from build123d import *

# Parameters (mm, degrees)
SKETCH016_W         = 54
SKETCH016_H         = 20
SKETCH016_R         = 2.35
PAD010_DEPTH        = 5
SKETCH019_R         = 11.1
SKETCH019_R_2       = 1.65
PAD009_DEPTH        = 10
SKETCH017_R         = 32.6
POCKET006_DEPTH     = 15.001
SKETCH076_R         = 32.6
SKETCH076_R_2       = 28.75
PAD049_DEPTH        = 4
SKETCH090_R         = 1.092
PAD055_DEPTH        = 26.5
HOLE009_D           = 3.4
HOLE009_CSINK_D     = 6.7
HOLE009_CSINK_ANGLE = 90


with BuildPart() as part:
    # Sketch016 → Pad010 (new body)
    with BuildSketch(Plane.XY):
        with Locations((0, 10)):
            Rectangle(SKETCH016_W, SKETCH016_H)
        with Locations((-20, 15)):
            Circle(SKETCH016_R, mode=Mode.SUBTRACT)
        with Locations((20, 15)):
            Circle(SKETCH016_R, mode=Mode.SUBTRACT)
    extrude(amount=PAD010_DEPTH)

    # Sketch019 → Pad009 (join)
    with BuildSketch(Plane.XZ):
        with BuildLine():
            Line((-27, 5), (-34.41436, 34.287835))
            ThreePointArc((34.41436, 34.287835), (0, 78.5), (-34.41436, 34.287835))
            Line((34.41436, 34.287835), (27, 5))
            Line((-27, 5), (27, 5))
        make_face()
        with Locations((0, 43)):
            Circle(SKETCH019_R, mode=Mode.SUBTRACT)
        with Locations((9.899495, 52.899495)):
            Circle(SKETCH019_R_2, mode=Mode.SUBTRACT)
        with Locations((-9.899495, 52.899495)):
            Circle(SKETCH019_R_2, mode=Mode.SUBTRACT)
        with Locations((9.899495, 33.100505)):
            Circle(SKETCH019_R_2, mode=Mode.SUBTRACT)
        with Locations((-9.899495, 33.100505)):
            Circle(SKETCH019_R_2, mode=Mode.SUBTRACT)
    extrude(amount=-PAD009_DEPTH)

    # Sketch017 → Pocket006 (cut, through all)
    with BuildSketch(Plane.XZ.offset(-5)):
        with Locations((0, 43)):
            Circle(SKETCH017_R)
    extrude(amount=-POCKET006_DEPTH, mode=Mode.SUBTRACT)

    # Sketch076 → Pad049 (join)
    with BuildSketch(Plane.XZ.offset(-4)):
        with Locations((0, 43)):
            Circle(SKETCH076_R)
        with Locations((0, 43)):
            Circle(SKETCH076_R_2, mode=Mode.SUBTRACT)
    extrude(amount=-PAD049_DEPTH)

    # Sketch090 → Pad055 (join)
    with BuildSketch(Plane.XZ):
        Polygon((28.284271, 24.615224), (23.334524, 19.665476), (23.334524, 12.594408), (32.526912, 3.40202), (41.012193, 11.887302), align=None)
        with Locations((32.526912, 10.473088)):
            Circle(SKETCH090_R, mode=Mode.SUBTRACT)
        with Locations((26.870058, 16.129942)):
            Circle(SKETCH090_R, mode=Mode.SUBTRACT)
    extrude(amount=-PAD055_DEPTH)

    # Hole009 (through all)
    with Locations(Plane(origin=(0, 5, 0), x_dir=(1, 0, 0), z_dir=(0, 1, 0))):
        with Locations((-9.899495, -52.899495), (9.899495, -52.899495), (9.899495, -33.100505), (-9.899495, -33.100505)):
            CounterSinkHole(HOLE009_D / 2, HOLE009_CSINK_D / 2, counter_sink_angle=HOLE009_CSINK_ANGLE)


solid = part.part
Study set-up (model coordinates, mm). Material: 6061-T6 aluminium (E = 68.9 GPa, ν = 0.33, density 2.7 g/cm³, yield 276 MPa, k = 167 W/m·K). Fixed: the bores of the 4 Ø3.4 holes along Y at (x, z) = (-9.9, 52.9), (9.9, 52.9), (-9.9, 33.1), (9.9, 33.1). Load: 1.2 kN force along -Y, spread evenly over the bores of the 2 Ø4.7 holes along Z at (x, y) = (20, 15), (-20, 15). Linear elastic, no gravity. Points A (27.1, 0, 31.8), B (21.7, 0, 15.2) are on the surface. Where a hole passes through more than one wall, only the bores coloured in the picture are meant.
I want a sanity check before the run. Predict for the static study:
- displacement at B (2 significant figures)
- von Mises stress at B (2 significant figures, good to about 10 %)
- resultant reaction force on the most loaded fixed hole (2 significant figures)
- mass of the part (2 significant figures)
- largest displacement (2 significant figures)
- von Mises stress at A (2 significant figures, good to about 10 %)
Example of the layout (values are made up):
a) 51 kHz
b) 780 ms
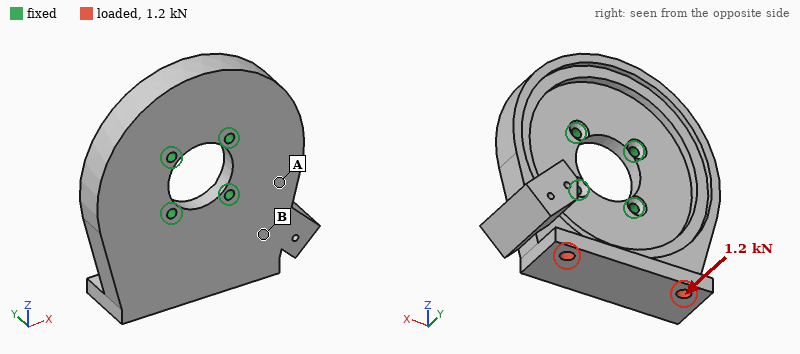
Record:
a) 0.12 mm
b) 20 MPa
c) 1.3 kN
d) 100 g
e) 0.27 mm
f) 55 MPa
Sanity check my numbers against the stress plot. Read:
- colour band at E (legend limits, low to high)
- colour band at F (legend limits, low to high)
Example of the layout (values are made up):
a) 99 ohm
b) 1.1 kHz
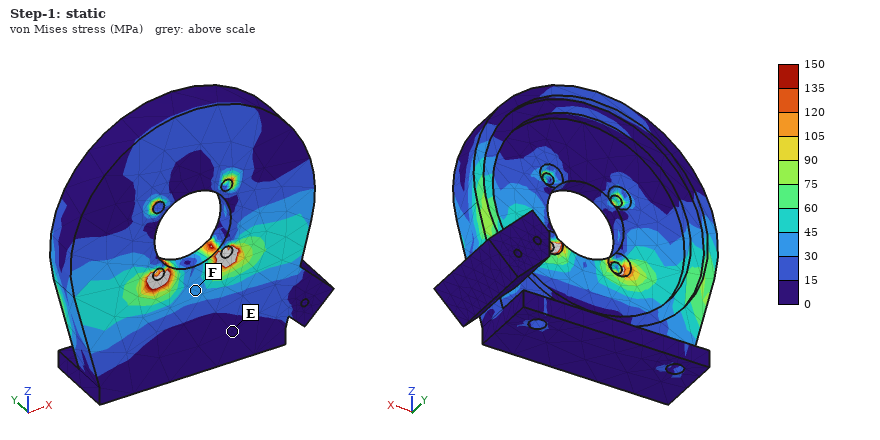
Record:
a) 0 to 15 MPa
b) 30 to 45 MPa
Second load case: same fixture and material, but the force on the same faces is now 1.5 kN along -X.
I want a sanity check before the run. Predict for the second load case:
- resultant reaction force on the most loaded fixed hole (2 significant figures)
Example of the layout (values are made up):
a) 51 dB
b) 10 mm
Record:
a) 1.6 kN
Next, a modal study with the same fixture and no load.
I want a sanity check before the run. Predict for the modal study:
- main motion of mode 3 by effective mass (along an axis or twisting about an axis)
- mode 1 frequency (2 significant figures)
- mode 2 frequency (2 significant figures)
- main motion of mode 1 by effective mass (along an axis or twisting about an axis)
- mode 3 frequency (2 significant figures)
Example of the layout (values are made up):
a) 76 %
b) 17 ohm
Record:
a) along Y
b) 1900 Hz
c) 2800 Hz
d) along Y
e) 5400 Hz
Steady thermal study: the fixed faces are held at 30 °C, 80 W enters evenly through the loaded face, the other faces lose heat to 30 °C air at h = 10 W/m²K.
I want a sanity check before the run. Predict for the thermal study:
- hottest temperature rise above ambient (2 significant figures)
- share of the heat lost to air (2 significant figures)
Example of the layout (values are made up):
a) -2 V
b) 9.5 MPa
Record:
a) 72 K
b) 4.1 %
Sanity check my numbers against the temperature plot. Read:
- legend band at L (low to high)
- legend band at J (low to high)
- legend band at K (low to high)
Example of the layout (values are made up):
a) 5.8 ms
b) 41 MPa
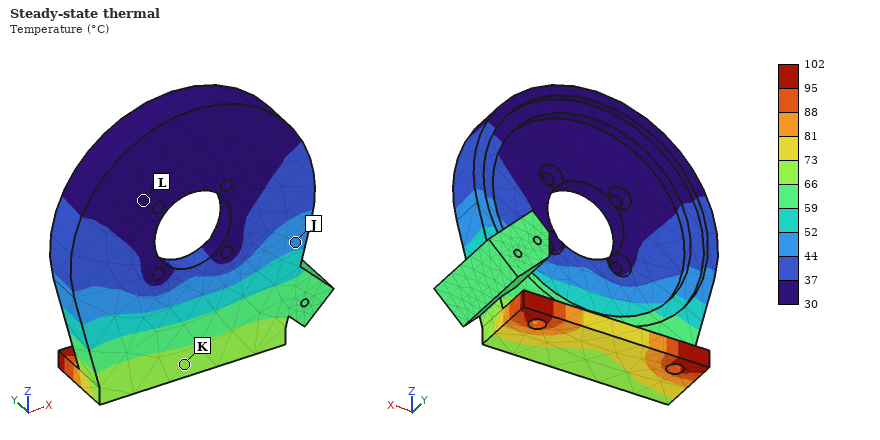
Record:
a) 30 to 37 °C
b) 44 to 52 °C
c) 66 to 73 °C
